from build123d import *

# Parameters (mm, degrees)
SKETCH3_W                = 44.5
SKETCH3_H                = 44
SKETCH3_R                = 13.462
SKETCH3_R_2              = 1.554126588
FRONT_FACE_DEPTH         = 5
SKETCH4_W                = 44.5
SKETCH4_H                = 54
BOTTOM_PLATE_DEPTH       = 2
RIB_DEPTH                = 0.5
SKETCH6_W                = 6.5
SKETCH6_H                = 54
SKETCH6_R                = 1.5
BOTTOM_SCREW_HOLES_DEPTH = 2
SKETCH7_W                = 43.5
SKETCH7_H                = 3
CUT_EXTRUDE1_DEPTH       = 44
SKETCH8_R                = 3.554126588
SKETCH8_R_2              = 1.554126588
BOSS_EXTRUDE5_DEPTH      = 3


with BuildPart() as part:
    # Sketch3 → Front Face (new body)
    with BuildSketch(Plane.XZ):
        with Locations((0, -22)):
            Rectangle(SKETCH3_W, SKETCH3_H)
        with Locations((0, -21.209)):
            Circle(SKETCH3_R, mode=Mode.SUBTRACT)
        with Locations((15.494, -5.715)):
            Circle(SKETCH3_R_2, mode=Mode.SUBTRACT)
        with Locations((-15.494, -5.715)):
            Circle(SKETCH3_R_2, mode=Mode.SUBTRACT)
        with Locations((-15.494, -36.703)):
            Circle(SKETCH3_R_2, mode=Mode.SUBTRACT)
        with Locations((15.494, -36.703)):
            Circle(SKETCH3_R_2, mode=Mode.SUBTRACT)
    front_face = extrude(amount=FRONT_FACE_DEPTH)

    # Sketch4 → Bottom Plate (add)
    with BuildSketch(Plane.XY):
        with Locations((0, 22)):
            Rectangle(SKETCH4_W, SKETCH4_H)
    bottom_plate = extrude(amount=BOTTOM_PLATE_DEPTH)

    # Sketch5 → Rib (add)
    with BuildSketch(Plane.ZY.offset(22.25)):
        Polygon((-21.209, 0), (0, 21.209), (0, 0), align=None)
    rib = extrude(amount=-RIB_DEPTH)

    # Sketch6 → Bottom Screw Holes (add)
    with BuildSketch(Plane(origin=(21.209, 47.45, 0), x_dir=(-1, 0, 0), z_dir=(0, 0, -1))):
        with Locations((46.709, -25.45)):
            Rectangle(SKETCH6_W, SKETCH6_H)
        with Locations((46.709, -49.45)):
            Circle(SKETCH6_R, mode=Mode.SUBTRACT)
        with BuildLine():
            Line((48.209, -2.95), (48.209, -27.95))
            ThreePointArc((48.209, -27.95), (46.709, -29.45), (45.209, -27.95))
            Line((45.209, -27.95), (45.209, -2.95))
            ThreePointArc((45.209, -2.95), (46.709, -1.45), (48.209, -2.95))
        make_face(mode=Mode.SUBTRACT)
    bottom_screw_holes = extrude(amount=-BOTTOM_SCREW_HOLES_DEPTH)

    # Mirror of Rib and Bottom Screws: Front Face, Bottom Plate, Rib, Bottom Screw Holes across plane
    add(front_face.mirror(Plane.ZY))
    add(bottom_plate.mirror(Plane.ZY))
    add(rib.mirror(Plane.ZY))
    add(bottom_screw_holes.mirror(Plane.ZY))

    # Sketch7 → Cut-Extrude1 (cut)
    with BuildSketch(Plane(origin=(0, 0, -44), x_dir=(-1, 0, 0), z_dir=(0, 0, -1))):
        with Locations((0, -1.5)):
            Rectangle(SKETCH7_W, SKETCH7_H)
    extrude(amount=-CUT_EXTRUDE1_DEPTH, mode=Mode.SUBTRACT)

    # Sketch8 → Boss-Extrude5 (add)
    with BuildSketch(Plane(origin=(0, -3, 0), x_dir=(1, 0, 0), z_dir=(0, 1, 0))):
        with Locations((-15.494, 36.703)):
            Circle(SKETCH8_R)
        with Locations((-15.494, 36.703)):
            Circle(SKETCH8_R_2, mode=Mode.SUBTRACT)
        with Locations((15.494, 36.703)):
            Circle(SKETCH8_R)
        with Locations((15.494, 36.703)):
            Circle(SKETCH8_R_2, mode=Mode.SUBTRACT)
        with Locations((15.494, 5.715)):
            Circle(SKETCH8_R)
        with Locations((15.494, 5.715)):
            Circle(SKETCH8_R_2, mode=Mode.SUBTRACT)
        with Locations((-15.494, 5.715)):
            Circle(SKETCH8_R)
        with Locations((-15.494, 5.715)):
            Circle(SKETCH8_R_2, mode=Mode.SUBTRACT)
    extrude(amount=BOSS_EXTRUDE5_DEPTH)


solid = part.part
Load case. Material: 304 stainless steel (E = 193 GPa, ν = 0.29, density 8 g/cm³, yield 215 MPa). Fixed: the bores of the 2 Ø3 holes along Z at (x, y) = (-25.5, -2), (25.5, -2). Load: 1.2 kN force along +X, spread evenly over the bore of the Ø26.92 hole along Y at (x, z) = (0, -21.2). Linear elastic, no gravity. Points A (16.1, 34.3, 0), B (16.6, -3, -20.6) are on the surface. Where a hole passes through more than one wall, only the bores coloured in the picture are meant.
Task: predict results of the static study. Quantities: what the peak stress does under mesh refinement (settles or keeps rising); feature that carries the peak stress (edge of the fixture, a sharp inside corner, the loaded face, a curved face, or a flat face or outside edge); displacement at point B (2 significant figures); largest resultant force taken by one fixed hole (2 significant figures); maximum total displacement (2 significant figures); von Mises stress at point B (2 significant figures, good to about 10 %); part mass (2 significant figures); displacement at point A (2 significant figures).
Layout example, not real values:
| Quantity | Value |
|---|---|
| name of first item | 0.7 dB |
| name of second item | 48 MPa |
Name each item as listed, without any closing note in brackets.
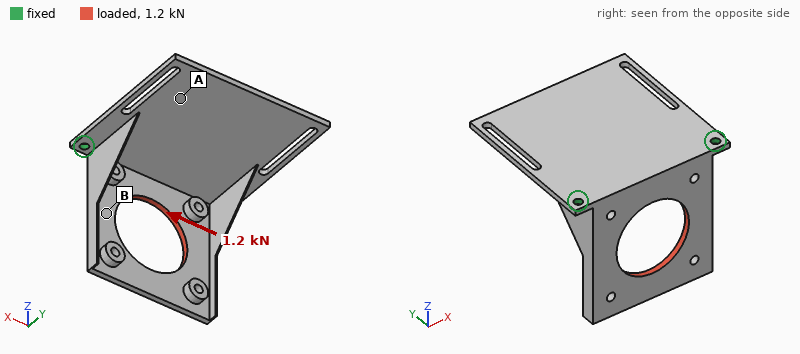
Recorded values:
| Quantity | Value |
|---|---|
| what the peak stress does under mesh refinement | keeps rising |
| feature that carries the peak stress | edge of the fixture |
| displacement at point B | 30 µm |
| largest resultant force taken by one fixed hole | 840 N |
| maximum total displacement | 66 µm |
| von Mises stress at point B | 59 MPa |
| part mass | 74 g |
| displacement at point A | 14 µm |
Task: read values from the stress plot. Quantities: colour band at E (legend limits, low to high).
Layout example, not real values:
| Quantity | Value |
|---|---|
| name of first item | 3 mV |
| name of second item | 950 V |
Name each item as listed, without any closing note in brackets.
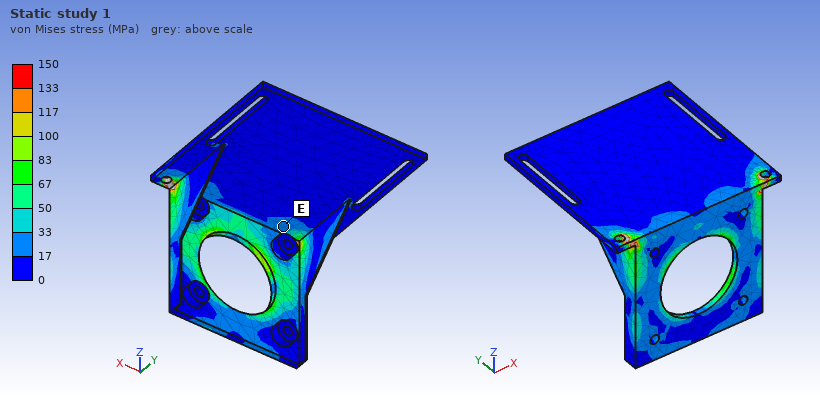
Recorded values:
| Quantity | Value |
|---|---|
| colour band at E | 17 to 33 MPa |
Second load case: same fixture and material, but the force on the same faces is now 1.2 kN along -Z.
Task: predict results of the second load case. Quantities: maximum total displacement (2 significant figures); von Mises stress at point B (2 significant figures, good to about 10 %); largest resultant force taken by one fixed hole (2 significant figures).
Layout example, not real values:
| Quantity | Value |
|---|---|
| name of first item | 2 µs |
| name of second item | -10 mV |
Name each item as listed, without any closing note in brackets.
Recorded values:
| Quantity | Value |
|---|---|
| maximum total displacement | 0.11 mm |
| von Mises stress at point B | 25 MPa |
| largest resultant force taken by one fixed hole | 680 N |
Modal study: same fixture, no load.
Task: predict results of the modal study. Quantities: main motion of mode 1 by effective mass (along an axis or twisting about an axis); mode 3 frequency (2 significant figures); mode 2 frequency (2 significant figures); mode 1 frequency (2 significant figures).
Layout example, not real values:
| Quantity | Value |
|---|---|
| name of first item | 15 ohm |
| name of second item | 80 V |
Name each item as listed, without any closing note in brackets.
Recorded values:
| Quantity | Value |
|---|---|
| main motion of mode 1 by effective mass | along Z |
| mode 3 frequency | 1600 Hz |
| mode 2 frequency | 1400 Hz |
| mode 1 frequency | 630 Hz |
